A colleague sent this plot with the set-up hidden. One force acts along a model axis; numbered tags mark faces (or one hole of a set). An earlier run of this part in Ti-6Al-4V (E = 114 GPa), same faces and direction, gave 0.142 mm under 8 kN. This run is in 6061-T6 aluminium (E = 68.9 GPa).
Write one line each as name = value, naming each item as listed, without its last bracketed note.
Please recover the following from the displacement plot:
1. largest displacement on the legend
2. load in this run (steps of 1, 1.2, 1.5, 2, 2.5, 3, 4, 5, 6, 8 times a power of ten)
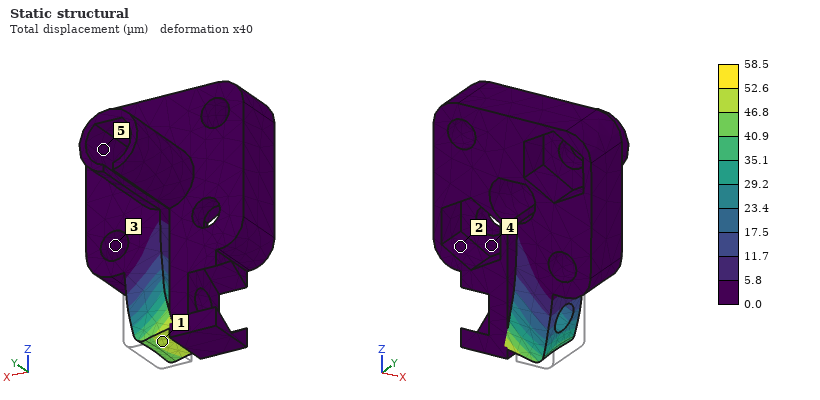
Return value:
largest displacement on the legend = 58.5 µm
load in this run = 2 kN
